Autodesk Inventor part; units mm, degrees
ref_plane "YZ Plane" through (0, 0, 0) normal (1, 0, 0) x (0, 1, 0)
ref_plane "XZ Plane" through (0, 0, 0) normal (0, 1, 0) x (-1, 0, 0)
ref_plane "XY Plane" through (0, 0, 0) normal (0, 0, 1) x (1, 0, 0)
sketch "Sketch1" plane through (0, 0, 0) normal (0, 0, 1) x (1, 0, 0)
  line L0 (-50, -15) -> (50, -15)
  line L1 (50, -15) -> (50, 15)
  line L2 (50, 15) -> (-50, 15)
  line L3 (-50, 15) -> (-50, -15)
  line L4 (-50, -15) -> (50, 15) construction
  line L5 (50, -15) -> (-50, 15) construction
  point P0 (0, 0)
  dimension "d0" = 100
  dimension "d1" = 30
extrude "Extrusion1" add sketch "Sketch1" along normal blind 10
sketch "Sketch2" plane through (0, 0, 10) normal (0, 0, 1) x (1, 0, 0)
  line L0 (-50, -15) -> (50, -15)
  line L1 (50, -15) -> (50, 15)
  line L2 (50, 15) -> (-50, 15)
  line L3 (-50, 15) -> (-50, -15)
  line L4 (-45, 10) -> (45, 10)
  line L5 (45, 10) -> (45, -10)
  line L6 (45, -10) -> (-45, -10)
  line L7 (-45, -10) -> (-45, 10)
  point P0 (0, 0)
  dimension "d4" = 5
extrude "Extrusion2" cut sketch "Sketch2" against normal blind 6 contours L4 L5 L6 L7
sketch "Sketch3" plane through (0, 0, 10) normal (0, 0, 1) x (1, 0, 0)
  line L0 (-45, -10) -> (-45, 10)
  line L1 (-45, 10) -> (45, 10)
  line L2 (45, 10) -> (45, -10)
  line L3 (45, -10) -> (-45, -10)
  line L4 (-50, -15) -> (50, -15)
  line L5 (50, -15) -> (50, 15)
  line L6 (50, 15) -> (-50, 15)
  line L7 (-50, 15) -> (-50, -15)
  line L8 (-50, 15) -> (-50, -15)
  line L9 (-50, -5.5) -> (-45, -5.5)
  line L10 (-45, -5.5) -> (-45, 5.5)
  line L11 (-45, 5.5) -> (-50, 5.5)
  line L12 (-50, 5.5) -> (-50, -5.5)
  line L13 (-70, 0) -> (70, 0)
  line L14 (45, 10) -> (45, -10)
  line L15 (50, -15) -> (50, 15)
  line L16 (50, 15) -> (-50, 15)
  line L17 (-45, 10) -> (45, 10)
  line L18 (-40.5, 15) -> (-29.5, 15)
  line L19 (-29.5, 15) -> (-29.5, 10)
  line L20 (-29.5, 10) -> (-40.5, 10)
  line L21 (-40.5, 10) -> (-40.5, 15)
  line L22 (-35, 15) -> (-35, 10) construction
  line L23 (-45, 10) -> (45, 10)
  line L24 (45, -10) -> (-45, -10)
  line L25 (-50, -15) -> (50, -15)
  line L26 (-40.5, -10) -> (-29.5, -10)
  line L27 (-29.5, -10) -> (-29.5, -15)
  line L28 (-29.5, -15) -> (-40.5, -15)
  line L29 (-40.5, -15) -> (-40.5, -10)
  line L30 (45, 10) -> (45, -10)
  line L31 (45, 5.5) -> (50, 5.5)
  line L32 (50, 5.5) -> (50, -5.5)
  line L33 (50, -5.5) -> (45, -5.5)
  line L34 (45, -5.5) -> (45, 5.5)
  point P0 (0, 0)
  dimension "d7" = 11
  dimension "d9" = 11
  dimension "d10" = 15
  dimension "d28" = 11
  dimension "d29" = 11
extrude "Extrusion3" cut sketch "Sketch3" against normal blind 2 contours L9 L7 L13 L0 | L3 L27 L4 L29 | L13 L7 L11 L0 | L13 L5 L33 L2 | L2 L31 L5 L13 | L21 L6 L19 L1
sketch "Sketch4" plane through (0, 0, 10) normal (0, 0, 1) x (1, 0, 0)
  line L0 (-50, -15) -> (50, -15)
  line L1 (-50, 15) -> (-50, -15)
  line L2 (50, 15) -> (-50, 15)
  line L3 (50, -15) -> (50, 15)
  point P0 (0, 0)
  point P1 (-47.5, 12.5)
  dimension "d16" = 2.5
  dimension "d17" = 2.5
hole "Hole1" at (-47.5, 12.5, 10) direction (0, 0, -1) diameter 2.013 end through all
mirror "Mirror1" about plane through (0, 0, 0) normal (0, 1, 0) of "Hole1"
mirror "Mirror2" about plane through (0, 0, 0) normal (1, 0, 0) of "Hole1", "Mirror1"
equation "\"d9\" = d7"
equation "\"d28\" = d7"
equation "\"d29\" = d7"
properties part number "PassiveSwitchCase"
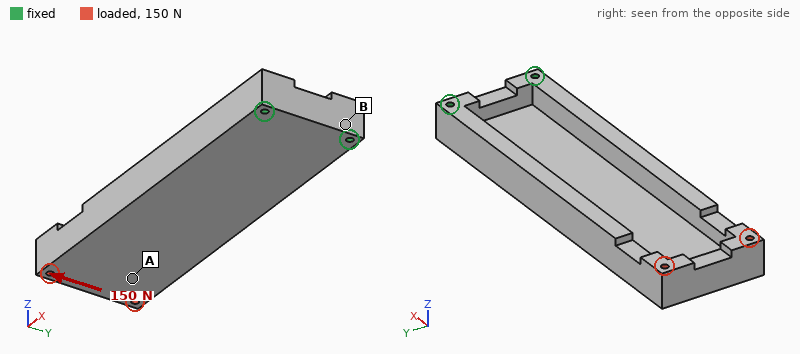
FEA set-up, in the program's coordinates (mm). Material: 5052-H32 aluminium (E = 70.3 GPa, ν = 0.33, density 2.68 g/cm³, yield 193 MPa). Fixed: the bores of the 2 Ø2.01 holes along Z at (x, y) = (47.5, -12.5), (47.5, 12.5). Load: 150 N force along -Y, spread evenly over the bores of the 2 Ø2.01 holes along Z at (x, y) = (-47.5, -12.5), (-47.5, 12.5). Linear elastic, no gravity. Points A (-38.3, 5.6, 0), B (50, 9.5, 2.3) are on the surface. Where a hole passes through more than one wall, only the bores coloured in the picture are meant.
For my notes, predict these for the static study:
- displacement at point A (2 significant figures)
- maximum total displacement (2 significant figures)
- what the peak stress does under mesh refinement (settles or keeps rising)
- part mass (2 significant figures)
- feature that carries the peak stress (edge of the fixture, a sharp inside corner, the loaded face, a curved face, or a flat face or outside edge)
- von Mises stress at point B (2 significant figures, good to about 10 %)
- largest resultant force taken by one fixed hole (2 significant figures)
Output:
35 µm
66 µm
keeps rising
50 g
edge of the fixture
2.7 MPa
560 N
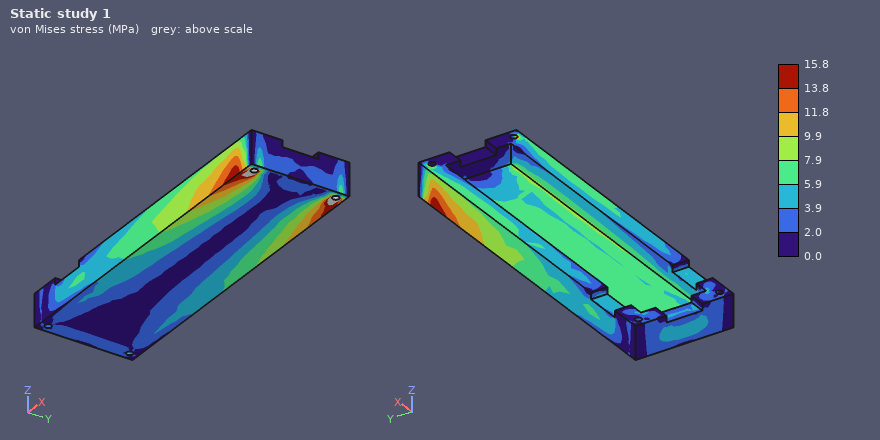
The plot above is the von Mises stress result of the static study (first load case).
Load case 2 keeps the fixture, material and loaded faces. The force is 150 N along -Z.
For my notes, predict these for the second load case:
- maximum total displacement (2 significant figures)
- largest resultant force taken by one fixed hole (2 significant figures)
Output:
0.52 mm
230 N
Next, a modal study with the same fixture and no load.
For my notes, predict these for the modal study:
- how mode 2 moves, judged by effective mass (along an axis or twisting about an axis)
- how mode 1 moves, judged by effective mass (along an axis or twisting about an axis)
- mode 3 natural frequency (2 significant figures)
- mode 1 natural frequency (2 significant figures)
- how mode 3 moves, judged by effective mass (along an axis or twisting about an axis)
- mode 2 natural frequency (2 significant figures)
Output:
along Y
along Z
3100 Hz
760 Hz
along Y
2100 Hz
